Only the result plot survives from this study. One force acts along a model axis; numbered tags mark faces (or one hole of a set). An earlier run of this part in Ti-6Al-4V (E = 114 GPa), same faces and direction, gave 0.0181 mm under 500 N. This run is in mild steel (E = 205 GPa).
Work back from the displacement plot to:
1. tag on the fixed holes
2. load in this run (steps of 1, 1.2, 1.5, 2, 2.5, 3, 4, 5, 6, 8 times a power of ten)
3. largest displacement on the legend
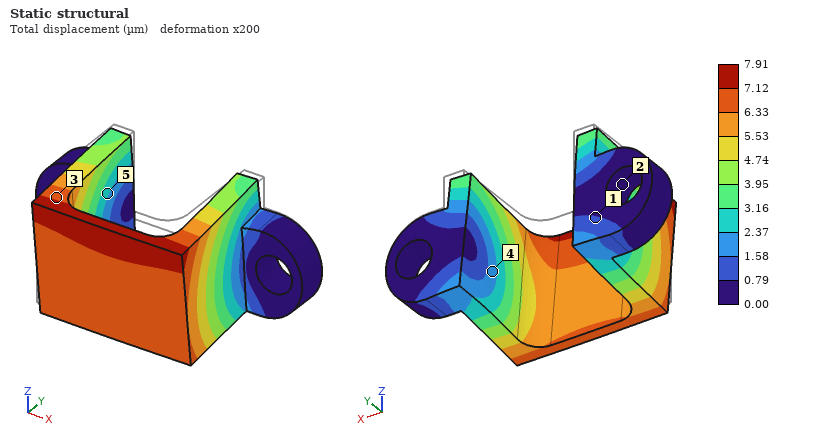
2
400 N
7.91 µm
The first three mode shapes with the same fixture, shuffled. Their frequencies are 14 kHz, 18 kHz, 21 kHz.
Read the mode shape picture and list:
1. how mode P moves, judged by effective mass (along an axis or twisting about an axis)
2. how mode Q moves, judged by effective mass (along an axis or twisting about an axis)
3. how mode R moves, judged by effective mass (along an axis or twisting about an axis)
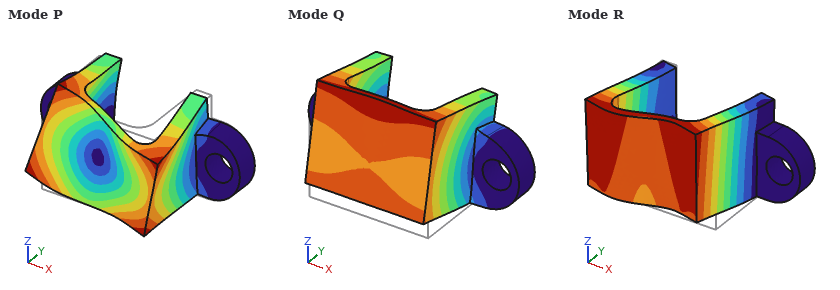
twisting about Y
along Z
along X
